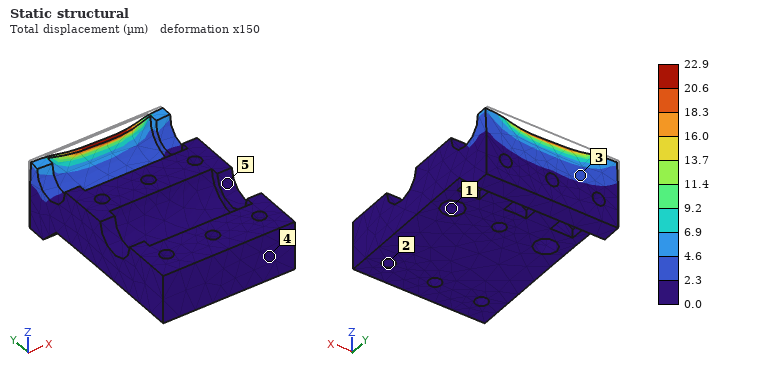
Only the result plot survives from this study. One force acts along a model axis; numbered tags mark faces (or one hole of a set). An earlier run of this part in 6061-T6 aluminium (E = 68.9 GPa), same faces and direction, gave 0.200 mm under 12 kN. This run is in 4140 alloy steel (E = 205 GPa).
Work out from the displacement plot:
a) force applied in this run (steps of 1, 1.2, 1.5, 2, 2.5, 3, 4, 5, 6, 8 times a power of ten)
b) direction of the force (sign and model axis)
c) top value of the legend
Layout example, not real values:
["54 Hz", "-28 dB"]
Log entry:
["4 kN", "-Y", "22.9 µm"]
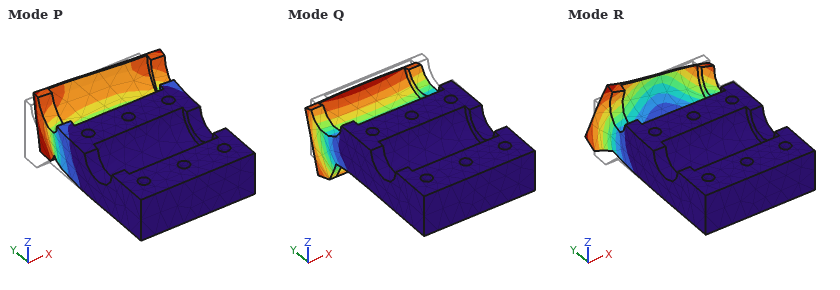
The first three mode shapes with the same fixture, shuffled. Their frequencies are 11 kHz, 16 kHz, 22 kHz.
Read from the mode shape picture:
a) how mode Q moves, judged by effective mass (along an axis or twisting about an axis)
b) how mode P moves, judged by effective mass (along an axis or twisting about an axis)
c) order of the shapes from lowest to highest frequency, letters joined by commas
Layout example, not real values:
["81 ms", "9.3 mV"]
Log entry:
["along Z", "along X", "Q, R, P"]
